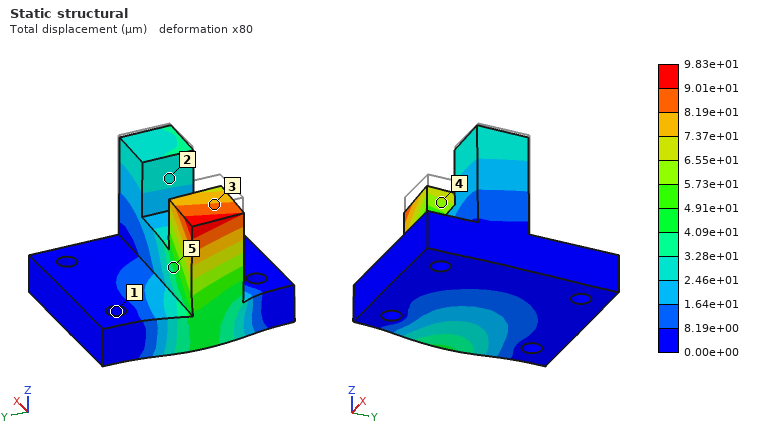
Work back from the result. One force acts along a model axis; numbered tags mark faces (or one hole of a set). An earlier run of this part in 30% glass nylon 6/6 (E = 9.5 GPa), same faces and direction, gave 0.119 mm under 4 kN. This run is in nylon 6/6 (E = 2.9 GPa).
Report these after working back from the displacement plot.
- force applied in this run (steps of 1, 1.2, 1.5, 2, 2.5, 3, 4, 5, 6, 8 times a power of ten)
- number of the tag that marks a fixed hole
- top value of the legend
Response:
1 kN
1
9.83e+01 µm
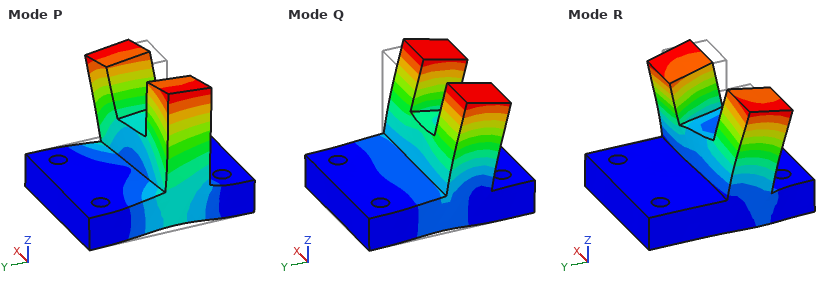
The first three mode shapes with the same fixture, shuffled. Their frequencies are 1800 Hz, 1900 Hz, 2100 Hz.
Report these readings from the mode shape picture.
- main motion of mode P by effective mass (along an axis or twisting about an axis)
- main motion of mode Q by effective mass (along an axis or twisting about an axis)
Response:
along X
along Y
